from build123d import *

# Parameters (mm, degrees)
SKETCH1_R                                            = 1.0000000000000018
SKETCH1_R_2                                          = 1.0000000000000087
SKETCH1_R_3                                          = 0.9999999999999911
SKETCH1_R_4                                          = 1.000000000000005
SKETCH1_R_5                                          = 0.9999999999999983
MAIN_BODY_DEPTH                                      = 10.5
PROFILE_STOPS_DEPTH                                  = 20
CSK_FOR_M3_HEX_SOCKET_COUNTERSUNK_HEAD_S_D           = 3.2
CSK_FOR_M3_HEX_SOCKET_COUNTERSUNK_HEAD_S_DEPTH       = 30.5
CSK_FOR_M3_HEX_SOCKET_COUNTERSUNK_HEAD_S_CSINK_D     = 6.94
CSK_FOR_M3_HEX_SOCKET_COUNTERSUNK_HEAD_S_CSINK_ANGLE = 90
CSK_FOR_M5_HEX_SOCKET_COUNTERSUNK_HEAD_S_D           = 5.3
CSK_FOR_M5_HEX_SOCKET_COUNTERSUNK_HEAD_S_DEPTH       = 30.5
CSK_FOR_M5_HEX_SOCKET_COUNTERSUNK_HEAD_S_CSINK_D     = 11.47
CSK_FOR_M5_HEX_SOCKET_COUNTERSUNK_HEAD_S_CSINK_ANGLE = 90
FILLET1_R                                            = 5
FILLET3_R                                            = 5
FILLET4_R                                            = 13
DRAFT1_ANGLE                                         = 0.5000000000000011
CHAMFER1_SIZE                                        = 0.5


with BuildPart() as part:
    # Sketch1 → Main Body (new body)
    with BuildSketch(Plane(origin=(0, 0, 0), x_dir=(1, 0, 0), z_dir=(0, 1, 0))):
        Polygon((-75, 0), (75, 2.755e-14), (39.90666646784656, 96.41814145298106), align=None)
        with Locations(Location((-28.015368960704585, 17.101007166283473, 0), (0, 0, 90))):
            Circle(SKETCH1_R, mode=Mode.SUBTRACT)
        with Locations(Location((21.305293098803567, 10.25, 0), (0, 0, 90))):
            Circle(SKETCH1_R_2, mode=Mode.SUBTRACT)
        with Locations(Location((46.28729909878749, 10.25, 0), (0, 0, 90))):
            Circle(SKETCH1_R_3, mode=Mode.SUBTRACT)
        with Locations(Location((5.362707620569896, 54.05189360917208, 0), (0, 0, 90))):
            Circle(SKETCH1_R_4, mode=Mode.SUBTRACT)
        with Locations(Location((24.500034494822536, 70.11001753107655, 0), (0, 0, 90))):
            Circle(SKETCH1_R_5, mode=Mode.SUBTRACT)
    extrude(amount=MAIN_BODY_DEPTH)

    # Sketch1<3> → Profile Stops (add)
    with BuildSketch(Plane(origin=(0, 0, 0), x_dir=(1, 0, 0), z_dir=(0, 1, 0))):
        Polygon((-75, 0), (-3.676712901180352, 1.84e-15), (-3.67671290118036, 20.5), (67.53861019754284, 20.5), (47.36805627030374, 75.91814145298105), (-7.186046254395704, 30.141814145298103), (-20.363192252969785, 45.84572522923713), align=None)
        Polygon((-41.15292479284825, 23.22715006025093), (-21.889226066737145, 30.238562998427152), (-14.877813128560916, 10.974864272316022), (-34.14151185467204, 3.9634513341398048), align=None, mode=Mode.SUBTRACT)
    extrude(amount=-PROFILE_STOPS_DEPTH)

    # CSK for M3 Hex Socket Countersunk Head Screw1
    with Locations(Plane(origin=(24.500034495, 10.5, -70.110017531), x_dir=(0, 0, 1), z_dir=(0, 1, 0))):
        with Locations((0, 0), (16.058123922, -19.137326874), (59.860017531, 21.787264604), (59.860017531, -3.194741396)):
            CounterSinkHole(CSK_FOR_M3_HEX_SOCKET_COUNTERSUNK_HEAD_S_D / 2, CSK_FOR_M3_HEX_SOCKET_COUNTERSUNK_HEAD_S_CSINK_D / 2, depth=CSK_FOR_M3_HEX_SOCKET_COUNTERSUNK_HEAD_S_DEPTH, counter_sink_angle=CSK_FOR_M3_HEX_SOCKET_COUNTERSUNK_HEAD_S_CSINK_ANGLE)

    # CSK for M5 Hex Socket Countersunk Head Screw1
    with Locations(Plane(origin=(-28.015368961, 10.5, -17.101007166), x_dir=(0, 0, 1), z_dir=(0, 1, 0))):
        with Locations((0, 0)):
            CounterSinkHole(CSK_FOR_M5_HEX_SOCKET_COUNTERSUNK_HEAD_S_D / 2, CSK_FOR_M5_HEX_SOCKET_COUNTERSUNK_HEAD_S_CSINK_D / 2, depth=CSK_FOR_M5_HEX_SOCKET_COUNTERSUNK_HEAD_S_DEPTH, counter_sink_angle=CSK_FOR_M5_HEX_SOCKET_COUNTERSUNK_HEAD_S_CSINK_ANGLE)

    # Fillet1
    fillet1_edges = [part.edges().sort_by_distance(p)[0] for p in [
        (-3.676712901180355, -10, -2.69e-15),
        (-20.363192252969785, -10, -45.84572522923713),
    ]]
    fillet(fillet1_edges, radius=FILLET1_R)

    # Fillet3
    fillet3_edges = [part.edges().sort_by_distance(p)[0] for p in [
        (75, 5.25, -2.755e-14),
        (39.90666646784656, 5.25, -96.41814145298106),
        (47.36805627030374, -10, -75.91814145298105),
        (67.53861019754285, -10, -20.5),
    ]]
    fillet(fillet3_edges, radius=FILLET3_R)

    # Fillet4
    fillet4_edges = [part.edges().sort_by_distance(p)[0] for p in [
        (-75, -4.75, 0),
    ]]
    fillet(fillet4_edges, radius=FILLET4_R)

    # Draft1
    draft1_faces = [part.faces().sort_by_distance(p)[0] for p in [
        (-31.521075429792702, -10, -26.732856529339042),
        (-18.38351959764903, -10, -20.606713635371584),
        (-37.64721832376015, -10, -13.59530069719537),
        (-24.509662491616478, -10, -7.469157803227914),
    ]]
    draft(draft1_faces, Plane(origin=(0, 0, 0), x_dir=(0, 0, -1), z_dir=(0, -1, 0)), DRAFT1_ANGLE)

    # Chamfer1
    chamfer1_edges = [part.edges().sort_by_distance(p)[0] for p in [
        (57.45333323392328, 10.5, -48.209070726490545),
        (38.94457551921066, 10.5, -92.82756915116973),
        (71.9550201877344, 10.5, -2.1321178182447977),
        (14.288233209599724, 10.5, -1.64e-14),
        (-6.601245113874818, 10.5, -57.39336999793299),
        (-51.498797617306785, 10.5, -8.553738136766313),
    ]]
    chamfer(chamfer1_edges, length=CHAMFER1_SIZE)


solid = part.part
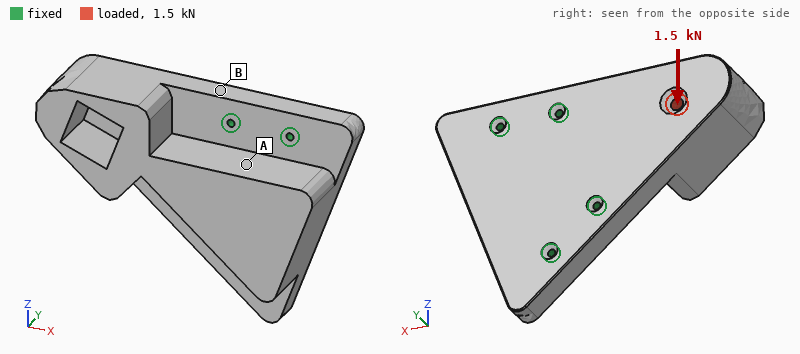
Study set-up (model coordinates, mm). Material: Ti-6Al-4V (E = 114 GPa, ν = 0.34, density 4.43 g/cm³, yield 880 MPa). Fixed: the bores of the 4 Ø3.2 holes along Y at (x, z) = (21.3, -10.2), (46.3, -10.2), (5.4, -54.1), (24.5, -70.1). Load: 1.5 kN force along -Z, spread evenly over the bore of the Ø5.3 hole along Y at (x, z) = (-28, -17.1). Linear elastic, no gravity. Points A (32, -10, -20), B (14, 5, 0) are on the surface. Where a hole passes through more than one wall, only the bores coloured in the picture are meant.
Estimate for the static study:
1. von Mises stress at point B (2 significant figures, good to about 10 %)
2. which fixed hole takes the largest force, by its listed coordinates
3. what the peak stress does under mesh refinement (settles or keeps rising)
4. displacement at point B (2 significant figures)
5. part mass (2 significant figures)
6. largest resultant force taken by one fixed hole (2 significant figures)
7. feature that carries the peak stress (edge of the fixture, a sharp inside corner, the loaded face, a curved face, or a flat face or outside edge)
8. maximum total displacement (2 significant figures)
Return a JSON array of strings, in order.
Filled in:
["5.7 MPa", "(5.4, -54.1)", "keeps rising", "1.2 µm", "620 g", "1.3 kN", "edge of the fixture", "6.9 µm"]
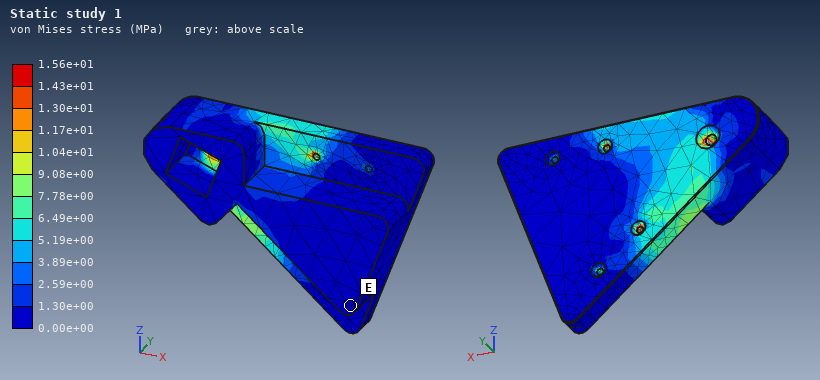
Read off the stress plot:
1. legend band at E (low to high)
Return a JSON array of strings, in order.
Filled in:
["0.00e+00 to 1.30e+00 MPa"]
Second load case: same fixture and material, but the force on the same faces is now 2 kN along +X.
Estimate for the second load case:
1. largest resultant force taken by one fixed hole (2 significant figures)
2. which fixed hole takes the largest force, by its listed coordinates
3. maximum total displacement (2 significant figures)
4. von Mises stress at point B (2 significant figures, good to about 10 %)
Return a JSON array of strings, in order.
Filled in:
["1.2 kN", "(21.3, -10.2)", "4.0 µm", "4.9 MPa"]
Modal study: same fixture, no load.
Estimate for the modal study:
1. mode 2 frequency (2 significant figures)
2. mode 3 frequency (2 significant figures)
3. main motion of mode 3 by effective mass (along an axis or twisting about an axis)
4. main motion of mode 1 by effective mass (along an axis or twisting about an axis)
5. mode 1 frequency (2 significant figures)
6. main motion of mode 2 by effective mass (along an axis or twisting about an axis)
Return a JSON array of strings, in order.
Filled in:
["6000 Hz", "6800 Hz", "along Y", "along Y", "2600 Hz", "along Z"]
